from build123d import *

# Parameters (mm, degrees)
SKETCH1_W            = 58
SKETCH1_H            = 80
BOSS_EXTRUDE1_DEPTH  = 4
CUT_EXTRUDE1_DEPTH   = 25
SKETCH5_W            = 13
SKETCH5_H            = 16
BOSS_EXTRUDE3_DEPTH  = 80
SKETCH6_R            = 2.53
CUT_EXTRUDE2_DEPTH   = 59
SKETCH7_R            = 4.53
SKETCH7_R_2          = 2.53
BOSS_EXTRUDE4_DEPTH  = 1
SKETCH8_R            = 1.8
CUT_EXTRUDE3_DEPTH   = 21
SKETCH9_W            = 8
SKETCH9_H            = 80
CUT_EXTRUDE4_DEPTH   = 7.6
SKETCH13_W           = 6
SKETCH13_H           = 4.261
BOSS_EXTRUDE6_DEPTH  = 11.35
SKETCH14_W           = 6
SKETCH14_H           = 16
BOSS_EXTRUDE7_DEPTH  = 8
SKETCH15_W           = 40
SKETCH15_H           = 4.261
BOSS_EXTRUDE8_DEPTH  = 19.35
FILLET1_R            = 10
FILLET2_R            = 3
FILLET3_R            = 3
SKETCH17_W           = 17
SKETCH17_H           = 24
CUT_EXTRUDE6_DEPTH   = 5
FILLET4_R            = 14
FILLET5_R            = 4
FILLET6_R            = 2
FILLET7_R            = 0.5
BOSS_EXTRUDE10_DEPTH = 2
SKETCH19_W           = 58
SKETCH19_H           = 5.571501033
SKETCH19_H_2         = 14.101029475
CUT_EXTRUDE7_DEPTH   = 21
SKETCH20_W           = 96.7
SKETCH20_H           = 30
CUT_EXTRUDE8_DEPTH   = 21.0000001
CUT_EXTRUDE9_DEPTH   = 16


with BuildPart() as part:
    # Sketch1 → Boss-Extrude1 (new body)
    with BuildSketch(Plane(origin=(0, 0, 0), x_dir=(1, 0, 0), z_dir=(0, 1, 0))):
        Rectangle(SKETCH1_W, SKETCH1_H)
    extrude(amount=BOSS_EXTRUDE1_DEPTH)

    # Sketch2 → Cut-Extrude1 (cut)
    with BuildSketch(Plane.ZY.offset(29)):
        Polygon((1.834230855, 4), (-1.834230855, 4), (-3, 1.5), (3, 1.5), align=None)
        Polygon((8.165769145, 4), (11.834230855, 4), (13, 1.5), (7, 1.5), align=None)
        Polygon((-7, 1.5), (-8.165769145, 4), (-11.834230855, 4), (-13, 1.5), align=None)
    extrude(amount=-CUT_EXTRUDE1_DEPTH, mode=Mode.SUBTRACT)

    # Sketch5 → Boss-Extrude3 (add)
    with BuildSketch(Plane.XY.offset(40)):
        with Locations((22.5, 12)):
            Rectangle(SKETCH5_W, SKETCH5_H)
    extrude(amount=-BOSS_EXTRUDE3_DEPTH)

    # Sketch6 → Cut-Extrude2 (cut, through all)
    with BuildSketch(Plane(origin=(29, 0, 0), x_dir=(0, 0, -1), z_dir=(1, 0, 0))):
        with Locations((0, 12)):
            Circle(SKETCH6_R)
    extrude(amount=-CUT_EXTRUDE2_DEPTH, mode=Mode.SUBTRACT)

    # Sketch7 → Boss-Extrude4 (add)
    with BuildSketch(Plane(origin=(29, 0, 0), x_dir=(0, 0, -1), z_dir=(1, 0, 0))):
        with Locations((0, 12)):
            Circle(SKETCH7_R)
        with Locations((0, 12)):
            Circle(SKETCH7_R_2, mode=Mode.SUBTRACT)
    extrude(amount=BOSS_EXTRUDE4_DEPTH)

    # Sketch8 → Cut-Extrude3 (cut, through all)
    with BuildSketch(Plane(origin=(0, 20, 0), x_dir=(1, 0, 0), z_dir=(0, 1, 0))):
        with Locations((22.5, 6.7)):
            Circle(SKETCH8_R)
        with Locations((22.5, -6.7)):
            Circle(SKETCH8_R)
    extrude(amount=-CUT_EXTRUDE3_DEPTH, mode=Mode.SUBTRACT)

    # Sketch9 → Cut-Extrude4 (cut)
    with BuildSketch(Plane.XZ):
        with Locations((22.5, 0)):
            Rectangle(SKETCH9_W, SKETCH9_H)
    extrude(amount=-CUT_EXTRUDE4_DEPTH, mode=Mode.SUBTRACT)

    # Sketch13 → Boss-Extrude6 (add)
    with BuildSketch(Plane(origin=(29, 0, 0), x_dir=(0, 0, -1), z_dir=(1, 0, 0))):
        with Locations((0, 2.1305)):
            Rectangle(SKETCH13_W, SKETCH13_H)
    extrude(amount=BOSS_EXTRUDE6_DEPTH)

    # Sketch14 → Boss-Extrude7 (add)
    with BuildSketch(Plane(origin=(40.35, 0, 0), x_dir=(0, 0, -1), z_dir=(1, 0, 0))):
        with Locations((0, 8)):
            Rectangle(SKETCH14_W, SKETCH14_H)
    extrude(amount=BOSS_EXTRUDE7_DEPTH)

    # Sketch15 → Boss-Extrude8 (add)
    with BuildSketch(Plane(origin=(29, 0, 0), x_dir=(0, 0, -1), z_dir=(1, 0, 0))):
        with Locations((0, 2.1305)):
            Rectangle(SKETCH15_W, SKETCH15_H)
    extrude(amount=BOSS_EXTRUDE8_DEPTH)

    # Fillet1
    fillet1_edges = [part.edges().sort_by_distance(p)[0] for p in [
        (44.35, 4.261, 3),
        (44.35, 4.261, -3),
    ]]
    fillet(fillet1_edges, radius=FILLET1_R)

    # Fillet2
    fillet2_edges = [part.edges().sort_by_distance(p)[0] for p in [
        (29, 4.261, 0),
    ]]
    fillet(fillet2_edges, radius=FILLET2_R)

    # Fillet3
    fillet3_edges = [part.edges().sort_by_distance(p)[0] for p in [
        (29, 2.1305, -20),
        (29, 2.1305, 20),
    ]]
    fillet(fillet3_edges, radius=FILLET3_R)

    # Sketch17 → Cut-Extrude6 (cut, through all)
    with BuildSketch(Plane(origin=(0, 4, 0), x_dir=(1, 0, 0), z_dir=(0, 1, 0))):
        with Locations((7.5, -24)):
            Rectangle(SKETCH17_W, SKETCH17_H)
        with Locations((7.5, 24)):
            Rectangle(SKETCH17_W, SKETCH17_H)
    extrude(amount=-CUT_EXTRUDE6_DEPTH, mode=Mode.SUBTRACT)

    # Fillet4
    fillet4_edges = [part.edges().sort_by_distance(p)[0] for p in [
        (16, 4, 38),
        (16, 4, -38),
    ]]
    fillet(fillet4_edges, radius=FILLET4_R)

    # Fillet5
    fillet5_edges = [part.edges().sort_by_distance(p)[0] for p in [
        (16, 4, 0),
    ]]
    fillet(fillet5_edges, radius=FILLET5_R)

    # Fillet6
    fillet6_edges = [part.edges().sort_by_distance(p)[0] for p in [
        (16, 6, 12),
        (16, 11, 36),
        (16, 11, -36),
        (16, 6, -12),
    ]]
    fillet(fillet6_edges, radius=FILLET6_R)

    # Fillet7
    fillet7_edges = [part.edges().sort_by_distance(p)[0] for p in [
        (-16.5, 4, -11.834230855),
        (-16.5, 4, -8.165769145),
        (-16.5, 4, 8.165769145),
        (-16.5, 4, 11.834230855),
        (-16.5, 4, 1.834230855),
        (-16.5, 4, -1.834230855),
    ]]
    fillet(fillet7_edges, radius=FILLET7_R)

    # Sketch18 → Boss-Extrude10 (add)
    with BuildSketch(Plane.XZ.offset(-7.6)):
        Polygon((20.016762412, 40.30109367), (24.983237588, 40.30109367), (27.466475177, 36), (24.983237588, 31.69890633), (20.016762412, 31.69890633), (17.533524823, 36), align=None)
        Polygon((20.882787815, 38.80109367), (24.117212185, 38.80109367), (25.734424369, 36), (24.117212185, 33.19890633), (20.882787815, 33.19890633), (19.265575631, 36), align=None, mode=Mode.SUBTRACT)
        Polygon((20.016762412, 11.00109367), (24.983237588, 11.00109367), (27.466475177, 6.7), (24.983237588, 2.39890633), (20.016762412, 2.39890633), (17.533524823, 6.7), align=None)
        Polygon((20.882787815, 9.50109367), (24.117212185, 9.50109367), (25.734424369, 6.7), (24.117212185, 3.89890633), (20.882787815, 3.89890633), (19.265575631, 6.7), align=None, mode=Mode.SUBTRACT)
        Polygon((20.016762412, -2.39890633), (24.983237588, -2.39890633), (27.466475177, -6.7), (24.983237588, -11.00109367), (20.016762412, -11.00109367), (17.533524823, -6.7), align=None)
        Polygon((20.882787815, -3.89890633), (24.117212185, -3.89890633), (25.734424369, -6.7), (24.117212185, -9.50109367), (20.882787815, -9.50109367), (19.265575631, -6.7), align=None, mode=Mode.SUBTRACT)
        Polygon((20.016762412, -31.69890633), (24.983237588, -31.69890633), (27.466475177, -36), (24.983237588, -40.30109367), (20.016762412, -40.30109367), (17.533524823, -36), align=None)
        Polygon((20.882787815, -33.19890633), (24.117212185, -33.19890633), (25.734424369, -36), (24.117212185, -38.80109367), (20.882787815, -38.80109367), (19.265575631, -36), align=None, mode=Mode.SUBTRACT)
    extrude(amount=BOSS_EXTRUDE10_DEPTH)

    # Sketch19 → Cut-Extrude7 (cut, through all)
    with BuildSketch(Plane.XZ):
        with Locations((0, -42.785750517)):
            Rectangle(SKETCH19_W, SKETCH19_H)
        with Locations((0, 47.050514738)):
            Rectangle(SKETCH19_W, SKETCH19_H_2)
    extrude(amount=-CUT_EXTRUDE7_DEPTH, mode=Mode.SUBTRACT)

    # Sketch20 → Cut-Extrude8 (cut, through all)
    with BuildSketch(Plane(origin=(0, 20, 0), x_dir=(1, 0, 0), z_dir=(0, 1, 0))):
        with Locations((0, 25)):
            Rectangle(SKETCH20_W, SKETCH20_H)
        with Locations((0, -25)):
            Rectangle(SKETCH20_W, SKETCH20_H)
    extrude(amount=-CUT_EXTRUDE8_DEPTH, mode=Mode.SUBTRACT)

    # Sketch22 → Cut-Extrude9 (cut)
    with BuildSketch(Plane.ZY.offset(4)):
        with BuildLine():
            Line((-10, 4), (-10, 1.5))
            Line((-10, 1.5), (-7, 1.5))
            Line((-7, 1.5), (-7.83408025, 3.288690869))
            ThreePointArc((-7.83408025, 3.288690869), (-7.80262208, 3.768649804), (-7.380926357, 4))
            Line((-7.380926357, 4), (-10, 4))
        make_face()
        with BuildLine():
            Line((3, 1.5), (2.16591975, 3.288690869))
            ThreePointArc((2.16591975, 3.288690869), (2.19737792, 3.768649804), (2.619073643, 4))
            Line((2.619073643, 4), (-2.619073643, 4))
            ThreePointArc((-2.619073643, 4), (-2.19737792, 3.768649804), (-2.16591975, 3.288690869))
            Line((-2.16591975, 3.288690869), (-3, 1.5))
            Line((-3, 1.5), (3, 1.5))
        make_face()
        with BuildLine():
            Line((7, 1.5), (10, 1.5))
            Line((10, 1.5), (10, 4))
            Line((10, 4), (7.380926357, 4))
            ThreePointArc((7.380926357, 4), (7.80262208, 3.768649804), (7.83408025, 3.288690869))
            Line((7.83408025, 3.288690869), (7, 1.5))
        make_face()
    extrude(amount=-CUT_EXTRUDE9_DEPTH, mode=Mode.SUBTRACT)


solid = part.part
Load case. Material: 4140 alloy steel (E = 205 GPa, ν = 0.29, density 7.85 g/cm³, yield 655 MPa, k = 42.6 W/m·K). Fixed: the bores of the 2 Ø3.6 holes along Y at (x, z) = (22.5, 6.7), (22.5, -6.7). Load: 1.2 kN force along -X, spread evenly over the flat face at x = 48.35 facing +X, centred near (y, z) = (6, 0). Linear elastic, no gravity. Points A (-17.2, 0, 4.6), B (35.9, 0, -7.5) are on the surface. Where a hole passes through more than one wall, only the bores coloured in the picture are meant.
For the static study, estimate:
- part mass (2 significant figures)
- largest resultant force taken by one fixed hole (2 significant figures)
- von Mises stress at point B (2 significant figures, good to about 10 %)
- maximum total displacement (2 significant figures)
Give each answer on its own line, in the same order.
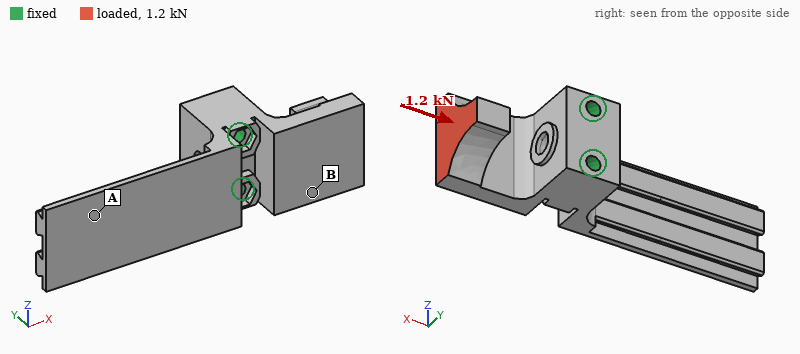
70 g
610 N
59 MPa
36 µm
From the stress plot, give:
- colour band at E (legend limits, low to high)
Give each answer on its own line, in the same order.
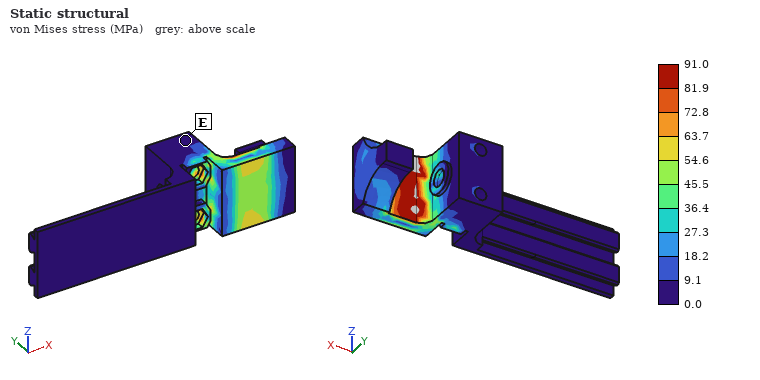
0.0 to 9.1 MPa
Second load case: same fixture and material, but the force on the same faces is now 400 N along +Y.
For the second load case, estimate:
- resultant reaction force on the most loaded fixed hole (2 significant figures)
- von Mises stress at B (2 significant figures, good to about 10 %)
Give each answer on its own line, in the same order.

210 N
82 MPa
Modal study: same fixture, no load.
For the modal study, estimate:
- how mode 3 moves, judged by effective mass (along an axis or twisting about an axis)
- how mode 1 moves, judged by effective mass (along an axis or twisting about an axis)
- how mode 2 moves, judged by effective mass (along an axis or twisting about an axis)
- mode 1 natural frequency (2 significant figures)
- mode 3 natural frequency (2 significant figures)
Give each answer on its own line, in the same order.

along Z
along Y
along Y
1300 Hz
3500 Hz
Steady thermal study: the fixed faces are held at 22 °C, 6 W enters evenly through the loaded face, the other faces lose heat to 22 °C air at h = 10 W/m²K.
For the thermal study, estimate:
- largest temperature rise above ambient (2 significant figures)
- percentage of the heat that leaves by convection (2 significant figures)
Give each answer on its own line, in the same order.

45 K
7.3 %
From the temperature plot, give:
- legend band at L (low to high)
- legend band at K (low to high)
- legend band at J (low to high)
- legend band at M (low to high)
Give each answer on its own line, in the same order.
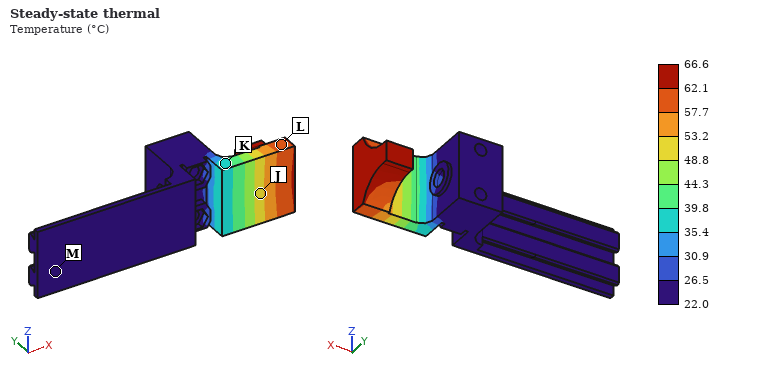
57.7 to 62.1 °C
35.4 to 39.8 °C
48.8 to 53.2 °C
22.0 to 26.5 °C
